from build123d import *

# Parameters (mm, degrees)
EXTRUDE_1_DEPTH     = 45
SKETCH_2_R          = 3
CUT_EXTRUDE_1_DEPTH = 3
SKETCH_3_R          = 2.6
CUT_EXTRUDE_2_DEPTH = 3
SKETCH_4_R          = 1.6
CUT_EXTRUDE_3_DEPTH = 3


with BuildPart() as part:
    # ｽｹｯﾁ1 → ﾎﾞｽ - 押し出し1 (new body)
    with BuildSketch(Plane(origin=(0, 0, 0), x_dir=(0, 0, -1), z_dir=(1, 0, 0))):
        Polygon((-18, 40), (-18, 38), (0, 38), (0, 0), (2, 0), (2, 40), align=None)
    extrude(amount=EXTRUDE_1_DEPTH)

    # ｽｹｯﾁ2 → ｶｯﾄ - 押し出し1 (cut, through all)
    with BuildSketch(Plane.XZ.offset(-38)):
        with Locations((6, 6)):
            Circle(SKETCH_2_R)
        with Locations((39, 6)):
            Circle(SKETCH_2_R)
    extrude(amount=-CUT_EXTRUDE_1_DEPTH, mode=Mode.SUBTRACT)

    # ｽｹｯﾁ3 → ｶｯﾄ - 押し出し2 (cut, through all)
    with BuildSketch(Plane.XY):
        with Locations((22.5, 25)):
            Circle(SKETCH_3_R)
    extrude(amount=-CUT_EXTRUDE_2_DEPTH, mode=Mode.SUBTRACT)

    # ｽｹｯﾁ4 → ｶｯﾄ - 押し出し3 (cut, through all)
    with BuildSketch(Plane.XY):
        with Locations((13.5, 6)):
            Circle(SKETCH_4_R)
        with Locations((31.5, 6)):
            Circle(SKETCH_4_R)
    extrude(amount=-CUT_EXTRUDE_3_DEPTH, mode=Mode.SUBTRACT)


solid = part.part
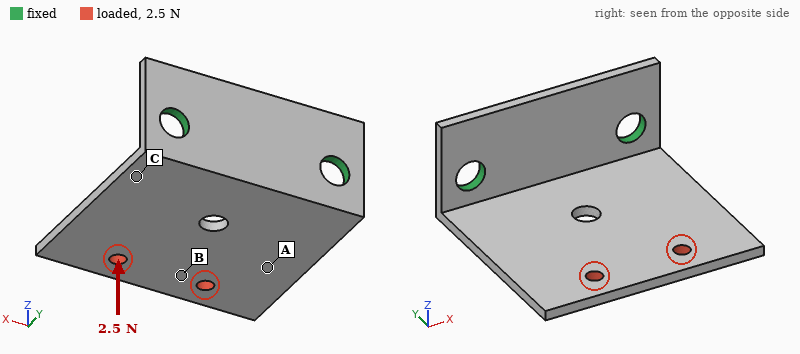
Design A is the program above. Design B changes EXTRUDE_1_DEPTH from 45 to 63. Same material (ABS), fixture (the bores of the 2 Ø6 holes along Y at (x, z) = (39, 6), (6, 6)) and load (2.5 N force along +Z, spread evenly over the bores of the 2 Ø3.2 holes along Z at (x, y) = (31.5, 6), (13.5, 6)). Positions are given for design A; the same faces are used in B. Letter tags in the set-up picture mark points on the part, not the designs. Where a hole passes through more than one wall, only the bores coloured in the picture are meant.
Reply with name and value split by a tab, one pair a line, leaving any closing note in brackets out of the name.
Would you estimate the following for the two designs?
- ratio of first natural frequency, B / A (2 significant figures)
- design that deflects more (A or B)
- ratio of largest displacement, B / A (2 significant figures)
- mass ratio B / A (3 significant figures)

ratio of first natural frequency, B / A	0.96
design that deflects more	A
ratio of largest displacement, B / A	0.82
mass ratio B / A	1.41
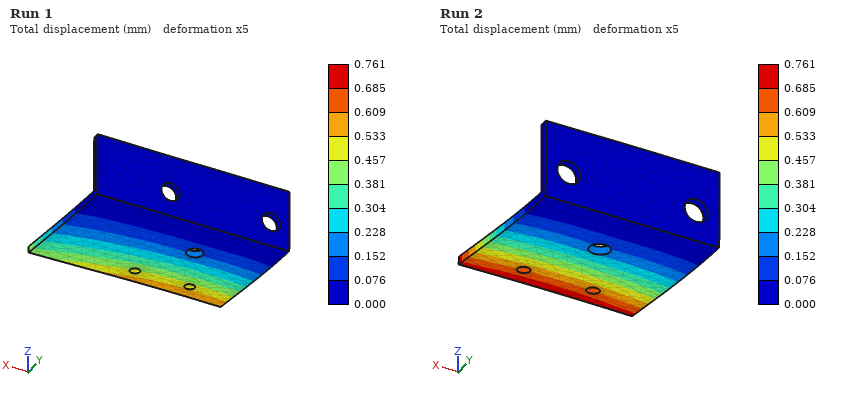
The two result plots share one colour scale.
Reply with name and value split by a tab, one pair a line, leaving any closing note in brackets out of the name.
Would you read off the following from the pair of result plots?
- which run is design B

which run is design B	Run 1
